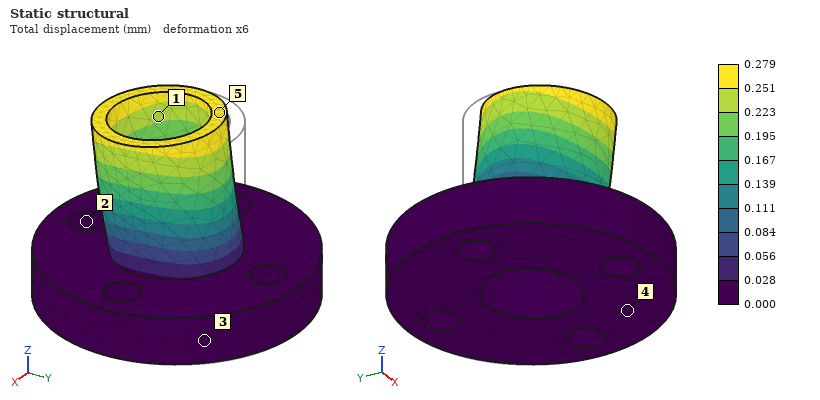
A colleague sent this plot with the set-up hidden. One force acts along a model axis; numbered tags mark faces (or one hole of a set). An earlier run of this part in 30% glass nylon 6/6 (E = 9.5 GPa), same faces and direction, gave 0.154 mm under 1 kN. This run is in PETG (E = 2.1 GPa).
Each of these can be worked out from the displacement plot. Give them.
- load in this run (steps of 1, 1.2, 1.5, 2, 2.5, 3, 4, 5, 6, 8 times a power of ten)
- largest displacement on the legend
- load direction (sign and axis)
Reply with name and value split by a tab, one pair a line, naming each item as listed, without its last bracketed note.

load in this run	400 N
largest displacement on the legend	0.279 mm
load direction	-Y
